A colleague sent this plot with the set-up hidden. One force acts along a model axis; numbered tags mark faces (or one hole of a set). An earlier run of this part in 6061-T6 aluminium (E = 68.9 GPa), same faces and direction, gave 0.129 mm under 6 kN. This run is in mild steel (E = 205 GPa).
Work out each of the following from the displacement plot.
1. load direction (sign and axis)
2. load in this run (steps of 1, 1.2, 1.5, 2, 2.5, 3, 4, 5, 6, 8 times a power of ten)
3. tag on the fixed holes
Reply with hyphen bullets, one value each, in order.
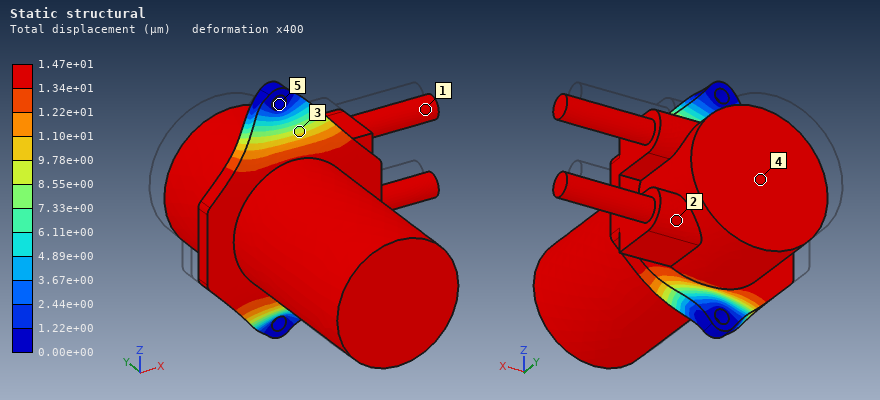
- -Y
- 2 kN
- 5
